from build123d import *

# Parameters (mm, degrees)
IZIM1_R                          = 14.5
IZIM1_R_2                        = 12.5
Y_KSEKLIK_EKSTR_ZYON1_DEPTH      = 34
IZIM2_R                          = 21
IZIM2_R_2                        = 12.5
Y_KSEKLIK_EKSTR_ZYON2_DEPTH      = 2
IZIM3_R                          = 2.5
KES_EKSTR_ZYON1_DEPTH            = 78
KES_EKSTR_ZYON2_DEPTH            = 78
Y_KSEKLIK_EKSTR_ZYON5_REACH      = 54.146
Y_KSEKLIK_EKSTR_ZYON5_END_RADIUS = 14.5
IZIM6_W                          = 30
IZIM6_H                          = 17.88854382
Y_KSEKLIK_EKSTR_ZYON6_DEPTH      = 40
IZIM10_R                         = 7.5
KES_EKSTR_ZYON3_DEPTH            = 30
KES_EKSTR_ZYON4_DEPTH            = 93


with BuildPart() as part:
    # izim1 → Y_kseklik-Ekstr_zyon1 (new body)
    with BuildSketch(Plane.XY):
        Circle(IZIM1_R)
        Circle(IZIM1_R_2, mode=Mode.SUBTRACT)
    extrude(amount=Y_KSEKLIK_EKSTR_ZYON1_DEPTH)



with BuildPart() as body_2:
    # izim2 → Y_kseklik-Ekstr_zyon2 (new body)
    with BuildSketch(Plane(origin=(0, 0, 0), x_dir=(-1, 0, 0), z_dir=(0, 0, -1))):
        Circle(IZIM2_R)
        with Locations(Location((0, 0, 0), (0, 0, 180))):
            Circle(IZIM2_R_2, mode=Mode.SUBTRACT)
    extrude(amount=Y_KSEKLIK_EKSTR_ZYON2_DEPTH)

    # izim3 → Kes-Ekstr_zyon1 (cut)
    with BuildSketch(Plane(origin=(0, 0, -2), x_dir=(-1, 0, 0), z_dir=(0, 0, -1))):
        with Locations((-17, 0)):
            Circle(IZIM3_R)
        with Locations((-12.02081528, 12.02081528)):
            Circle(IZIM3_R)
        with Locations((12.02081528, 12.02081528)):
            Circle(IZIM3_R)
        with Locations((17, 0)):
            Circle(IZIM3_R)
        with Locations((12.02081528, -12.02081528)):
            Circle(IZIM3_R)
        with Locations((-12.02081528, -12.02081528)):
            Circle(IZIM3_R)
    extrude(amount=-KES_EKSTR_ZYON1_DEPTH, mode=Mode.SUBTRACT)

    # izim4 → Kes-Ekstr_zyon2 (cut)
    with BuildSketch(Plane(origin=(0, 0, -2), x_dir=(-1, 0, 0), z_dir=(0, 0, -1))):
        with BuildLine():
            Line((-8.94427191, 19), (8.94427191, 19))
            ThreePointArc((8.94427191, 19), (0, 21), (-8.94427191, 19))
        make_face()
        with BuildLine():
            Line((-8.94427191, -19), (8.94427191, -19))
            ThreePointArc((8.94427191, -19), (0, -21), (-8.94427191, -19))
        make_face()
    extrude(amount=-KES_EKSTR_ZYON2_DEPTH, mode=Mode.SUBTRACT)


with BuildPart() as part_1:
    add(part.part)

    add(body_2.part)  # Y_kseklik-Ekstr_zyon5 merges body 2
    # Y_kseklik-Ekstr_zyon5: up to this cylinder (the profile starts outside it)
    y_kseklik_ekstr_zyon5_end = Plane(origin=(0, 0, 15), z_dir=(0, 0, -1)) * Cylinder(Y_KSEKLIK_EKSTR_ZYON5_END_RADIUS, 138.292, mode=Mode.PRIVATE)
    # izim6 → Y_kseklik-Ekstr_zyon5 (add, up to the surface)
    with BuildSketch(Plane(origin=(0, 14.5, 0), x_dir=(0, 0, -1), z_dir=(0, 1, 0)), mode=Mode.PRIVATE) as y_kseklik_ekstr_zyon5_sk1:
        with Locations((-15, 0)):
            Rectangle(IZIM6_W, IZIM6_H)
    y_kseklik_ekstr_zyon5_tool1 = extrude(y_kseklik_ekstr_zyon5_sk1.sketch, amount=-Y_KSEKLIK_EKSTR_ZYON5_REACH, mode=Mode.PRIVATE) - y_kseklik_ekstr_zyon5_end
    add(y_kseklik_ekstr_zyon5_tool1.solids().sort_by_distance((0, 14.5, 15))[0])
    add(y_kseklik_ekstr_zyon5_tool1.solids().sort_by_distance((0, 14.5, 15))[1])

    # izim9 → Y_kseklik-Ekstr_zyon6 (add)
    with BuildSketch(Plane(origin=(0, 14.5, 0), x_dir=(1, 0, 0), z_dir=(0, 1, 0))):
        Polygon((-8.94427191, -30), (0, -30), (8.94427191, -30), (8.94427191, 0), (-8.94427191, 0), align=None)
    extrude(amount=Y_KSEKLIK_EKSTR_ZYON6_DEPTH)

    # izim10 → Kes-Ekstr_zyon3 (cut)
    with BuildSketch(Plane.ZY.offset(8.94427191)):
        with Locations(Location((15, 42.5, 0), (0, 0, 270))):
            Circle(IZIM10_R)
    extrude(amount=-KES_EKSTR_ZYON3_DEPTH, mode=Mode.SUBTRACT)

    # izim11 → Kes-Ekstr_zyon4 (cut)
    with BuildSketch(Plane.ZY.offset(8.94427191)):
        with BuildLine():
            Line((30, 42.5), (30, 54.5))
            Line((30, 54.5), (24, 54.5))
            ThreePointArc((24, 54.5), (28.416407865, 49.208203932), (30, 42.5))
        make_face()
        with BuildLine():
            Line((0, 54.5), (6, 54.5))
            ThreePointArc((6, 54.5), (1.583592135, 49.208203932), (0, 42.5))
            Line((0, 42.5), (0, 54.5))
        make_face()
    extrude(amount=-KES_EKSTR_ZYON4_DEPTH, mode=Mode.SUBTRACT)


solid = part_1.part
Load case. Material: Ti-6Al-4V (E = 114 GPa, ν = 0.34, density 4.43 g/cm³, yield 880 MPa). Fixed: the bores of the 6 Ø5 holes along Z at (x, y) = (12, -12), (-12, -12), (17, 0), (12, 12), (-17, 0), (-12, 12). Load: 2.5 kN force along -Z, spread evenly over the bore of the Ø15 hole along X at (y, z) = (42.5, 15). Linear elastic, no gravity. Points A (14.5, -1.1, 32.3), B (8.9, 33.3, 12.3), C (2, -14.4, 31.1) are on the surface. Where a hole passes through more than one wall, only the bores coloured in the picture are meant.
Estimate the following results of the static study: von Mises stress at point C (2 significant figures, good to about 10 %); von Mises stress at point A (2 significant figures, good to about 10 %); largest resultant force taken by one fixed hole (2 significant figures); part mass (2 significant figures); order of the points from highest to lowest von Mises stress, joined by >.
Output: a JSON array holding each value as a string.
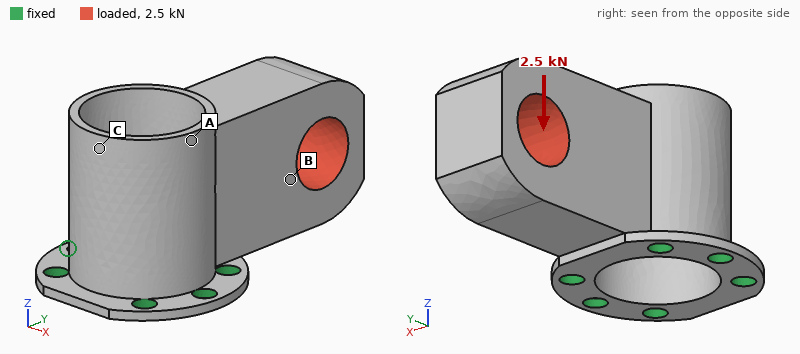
["64 MPa", "87 MPa", "3.5 kN", "110 g", "A > C > B"]
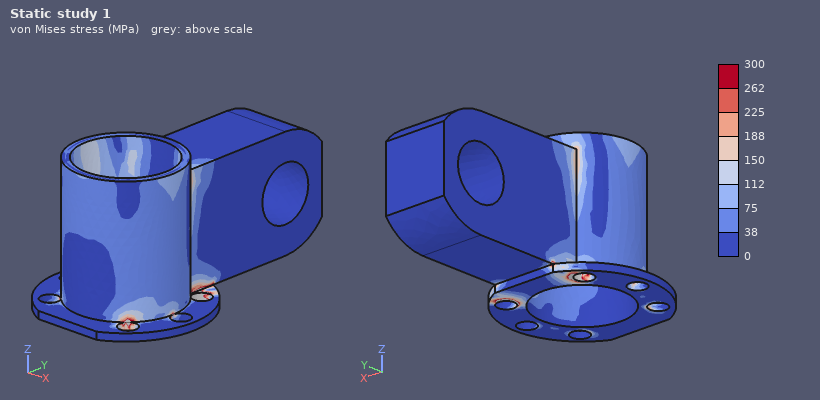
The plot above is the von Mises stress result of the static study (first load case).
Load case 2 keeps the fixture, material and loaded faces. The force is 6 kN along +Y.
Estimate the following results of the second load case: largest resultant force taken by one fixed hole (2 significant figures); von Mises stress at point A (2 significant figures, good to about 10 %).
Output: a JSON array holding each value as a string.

["2.9 kN", "97 MPa"]
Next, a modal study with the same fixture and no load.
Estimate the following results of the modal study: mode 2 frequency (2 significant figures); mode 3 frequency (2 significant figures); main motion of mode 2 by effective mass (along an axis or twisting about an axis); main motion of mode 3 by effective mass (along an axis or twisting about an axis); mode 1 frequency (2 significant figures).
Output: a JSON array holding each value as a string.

["4200 Hz", "7700 Hz", "along X", "along X", "3000 Hz"]
